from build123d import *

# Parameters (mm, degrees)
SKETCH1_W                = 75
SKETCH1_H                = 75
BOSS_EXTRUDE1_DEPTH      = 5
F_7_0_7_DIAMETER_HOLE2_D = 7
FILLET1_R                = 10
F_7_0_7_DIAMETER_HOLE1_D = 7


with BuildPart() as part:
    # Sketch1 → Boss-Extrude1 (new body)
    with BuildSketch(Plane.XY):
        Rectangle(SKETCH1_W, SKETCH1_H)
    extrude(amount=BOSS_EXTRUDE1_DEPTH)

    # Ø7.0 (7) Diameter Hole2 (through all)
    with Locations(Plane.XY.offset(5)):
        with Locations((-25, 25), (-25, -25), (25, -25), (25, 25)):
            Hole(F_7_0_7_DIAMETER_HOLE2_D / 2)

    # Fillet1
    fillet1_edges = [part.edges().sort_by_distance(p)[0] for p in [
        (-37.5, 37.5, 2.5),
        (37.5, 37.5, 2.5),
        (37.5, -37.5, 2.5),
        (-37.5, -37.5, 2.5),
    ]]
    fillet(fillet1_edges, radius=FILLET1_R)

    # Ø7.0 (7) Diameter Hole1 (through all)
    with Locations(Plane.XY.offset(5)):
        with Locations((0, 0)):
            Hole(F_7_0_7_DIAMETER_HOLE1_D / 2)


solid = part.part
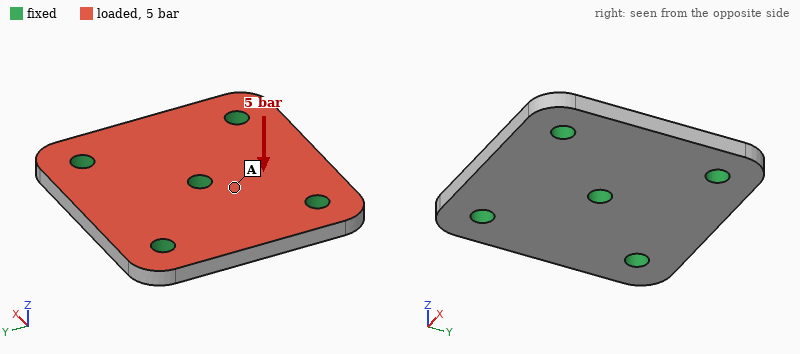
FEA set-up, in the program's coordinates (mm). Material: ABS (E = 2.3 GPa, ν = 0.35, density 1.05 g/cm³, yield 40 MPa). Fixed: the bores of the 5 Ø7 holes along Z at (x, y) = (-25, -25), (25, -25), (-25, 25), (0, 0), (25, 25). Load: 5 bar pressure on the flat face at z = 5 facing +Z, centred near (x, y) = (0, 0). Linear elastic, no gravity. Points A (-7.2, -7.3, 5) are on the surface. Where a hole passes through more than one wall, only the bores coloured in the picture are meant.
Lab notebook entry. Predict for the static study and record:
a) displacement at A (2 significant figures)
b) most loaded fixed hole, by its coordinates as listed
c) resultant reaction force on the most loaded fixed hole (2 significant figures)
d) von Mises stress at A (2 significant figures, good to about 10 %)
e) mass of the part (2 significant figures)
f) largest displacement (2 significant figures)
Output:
0.065 mm
(0, 0)
600 N
6.1 MPa
28 g
0.33 mm
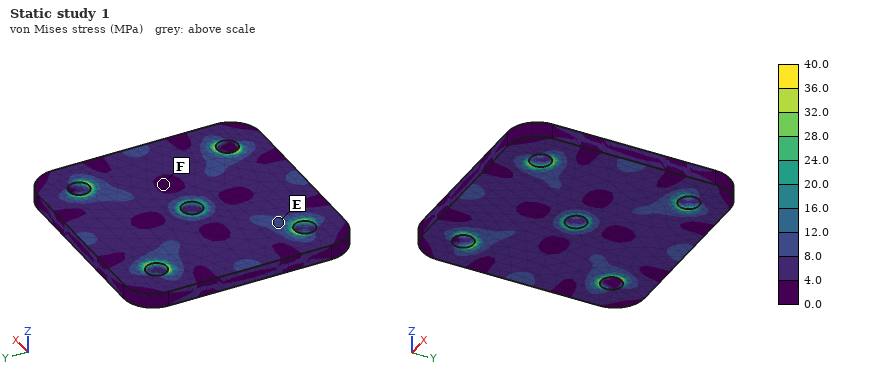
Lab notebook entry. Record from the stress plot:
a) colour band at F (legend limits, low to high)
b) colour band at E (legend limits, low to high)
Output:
0.0 to 4.0 MPa
8.0 to 12.0 MPa
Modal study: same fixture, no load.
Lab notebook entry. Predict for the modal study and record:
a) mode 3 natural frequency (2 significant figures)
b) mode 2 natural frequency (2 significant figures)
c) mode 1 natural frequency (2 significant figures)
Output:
3400 Hz
3400 Hz
3300 Hz
